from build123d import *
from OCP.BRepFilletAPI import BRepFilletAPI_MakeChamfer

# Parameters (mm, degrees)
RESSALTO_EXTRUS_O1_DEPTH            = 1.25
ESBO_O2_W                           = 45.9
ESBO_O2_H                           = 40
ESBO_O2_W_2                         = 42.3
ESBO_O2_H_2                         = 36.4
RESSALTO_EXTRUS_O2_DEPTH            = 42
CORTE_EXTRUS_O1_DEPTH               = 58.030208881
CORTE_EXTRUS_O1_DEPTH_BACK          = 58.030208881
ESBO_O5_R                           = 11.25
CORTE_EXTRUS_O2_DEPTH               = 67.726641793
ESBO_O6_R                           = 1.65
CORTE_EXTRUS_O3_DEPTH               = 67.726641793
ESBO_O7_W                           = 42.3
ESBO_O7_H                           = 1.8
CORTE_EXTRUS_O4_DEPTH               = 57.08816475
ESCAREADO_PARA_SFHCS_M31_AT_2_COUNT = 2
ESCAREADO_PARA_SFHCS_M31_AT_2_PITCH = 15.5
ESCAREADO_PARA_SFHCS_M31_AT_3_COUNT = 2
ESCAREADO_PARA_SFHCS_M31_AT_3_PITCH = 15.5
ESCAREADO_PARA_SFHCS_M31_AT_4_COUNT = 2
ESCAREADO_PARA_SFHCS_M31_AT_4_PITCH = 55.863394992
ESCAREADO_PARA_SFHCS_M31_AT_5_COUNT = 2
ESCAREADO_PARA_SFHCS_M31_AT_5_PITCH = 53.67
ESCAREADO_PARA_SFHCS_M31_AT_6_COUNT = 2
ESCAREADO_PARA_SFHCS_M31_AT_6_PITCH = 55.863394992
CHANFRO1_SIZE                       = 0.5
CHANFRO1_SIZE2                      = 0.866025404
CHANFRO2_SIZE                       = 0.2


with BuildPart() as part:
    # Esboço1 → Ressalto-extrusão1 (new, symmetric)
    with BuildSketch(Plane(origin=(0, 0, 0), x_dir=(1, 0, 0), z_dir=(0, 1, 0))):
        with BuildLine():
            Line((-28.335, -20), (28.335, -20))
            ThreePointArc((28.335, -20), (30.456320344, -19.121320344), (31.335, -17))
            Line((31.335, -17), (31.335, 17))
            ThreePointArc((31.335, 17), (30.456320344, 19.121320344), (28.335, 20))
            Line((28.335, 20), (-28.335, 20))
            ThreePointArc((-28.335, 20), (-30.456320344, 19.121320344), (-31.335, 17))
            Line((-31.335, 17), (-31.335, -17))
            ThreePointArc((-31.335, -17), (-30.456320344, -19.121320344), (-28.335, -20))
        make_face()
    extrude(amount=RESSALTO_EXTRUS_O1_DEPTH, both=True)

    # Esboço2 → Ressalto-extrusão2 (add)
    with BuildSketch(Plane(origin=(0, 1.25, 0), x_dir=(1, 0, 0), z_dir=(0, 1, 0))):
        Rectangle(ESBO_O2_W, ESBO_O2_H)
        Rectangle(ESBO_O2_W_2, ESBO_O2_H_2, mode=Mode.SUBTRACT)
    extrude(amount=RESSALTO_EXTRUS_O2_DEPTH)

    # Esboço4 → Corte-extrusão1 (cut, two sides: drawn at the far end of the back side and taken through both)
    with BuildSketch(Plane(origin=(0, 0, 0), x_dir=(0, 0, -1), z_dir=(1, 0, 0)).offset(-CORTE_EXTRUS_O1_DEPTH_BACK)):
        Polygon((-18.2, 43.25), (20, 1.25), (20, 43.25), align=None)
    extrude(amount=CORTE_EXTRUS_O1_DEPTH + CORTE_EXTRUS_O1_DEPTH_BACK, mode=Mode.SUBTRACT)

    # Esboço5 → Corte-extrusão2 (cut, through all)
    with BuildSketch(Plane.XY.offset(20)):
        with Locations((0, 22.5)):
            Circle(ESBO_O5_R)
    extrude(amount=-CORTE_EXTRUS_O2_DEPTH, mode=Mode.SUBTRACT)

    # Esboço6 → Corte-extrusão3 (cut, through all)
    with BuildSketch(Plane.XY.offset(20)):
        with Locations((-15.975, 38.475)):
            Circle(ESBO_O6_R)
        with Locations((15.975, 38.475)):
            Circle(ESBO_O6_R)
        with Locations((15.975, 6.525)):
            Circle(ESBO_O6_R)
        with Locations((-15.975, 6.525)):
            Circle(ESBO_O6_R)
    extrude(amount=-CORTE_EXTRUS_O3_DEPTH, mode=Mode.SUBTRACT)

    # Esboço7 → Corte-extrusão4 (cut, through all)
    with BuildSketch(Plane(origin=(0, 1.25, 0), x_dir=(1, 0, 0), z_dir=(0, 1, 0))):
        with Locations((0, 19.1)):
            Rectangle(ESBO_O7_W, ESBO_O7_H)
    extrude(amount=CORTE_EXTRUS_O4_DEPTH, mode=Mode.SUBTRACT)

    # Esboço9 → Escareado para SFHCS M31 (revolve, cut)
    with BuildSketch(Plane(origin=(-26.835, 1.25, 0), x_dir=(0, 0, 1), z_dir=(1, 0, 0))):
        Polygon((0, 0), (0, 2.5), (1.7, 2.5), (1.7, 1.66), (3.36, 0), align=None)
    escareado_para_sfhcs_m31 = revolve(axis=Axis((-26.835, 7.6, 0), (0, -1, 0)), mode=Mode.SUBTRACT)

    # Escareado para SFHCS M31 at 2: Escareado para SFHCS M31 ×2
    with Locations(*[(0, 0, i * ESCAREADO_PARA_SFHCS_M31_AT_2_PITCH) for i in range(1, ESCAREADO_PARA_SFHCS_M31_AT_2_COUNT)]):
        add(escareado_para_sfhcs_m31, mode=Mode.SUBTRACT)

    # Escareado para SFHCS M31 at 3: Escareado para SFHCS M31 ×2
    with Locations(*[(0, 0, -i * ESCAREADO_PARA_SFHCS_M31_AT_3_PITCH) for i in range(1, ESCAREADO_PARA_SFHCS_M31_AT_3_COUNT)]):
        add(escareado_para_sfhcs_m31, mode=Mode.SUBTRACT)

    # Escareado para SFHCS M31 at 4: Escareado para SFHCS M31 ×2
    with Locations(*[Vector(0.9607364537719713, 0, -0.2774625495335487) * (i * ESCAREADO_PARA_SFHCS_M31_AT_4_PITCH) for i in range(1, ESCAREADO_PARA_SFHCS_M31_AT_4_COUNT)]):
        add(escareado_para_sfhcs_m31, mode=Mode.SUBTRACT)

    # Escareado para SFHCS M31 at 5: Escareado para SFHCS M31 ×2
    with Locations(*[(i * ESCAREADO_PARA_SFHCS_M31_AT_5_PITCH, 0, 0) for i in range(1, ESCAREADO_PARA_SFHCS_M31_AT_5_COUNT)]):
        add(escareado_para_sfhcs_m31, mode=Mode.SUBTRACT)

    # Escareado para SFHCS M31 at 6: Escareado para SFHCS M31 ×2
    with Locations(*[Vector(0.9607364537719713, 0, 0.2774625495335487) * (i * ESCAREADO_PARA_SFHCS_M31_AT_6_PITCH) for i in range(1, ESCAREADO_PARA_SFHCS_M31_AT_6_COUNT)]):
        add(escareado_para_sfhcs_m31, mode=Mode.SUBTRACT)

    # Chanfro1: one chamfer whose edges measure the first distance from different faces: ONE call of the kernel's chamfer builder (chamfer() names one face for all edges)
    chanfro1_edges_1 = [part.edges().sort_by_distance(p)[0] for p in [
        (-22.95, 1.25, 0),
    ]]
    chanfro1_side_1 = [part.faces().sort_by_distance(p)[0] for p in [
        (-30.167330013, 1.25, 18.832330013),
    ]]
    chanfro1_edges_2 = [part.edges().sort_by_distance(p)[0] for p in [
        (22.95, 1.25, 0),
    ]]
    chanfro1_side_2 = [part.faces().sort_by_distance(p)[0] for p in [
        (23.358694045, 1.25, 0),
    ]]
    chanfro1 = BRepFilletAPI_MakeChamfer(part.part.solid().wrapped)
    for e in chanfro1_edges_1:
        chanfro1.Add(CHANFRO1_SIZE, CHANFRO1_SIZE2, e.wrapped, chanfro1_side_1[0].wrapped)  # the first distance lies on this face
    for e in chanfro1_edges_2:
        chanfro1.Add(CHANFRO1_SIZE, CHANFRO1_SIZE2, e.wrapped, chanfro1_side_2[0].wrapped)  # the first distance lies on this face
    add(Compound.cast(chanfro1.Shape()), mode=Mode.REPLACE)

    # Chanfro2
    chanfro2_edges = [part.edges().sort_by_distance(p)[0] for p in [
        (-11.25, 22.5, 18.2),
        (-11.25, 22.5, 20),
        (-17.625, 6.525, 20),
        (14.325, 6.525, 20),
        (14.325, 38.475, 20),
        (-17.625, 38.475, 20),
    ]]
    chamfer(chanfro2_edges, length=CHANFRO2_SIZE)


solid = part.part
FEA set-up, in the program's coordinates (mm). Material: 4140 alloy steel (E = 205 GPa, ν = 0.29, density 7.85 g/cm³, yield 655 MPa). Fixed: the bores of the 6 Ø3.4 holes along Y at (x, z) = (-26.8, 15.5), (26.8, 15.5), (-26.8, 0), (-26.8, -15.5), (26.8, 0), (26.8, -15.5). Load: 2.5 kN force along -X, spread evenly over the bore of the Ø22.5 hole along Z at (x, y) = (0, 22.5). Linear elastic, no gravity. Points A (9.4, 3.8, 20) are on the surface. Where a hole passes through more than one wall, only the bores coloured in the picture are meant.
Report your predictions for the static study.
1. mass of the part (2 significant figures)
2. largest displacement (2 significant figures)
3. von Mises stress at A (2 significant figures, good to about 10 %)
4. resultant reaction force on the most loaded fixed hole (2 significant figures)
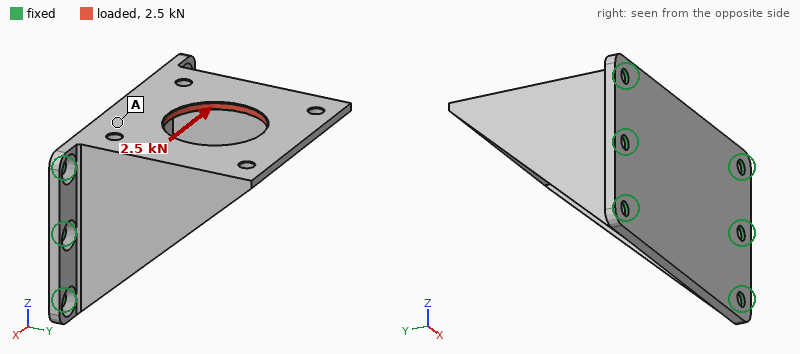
91 g
55 µm
42 MPa
1.5 kN
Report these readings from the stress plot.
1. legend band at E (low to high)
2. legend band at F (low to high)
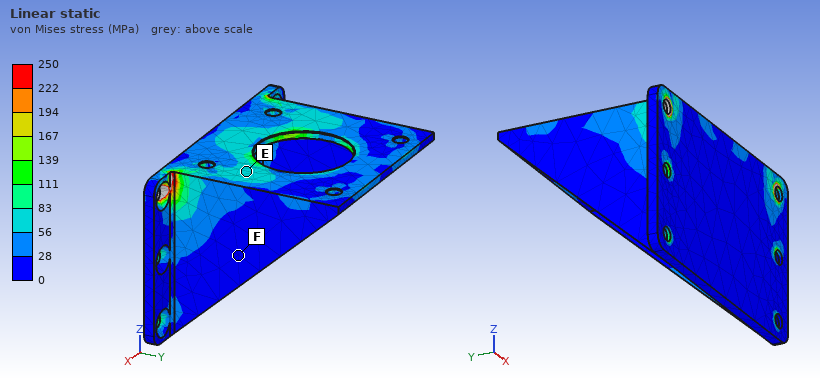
56 to 83 MPa
0 to 28 MPa
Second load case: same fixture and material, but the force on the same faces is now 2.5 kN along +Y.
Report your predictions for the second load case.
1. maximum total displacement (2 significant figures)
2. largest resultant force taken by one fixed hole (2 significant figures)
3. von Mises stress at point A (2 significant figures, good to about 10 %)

44 µm
1.6 kN
32 MPa
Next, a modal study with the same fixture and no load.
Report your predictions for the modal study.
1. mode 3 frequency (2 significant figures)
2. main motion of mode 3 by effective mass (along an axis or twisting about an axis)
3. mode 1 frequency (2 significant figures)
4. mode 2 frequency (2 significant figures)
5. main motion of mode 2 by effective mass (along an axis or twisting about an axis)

5300 Hz
along X
3100 Hz
4300 Hz
along Y
